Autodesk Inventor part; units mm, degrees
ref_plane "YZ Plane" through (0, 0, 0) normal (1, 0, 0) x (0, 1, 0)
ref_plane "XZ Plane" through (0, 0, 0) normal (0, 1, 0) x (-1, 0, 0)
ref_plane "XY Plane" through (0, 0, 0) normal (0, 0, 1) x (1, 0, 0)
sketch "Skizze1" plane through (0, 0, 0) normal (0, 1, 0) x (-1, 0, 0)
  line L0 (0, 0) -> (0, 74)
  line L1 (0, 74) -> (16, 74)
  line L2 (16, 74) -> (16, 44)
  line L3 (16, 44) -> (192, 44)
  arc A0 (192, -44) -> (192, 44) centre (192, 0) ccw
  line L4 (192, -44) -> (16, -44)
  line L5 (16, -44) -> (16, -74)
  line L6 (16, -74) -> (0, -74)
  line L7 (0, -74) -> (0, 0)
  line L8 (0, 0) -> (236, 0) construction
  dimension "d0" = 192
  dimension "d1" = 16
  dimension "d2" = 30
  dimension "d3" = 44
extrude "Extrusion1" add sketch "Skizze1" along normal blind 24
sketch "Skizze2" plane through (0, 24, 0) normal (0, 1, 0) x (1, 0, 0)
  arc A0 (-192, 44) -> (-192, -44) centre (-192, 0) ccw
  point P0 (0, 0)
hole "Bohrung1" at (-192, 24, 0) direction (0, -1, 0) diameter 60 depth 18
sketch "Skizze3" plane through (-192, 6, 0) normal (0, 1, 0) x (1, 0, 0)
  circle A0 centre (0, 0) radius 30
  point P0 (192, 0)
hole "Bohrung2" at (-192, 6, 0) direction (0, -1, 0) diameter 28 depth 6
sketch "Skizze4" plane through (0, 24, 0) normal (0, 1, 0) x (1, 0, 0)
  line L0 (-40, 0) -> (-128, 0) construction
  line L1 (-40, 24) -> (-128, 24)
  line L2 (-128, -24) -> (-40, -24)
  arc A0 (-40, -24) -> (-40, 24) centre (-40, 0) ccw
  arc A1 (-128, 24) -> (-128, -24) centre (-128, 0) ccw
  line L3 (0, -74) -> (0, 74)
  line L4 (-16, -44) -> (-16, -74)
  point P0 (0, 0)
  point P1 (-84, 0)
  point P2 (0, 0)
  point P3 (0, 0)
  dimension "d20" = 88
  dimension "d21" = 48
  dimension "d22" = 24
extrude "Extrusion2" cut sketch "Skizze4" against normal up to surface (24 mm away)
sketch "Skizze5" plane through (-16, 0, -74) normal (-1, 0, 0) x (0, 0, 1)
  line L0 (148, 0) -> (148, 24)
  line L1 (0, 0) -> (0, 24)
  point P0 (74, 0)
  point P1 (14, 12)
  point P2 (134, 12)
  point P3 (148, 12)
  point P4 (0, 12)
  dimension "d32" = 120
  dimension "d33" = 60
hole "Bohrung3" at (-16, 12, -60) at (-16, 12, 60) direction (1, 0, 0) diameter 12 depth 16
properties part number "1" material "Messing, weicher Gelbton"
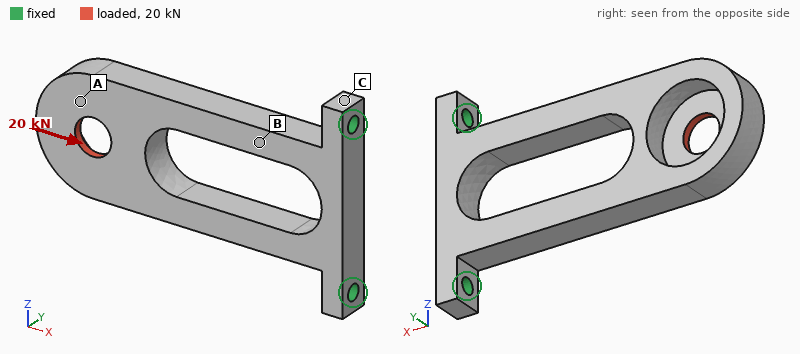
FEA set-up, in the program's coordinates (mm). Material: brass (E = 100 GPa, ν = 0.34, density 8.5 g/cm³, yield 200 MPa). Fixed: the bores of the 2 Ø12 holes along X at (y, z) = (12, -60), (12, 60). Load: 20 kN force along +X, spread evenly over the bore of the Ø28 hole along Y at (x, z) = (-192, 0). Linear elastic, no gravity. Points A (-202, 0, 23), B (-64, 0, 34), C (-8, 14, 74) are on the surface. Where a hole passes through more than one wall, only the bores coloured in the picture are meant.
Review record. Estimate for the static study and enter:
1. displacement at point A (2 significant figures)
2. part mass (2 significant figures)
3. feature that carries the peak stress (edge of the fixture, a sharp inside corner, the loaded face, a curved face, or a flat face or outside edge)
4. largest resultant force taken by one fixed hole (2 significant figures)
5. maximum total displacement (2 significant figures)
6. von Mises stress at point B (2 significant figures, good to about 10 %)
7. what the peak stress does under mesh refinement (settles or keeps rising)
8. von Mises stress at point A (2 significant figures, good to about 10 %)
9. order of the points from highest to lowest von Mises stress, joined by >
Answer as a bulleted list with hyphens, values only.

- 1.0 mm
- 2.5 kg
- edge of the fixture
- 10 kN
- 1.3 mm
- 68 MPa
- keeps rising
- 28 MPa
- B > A > C
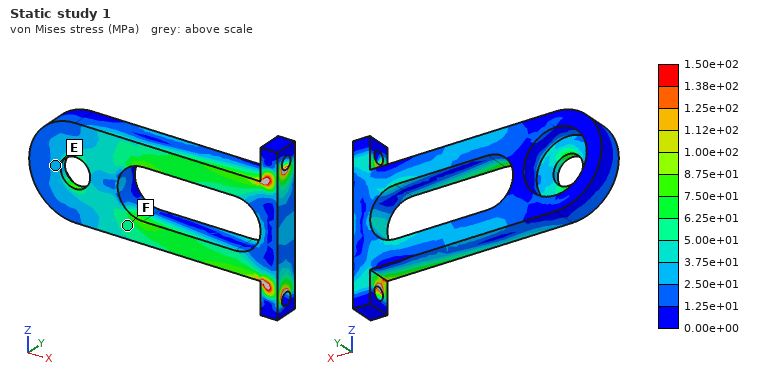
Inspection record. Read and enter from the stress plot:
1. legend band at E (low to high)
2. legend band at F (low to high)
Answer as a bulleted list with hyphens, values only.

- 2.50e+01 to 3.75e+01 MPa
- 5.00e+01 to 6.25e+01 MPa
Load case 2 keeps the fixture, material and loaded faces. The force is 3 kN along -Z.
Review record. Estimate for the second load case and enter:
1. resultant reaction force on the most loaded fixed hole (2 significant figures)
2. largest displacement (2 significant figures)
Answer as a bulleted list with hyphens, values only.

- 5.8 kN
- 0.31 mm
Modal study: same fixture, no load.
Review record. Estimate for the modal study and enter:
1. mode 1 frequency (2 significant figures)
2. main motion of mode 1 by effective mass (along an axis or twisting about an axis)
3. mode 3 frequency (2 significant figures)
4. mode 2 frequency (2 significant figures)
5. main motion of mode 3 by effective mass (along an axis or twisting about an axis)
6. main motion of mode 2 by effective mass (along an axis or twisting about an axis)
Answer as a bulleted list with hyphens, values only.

- 180 Hz
- along Y
- 740 Hz
- 480 Hz
- twisting about X
- along Z
